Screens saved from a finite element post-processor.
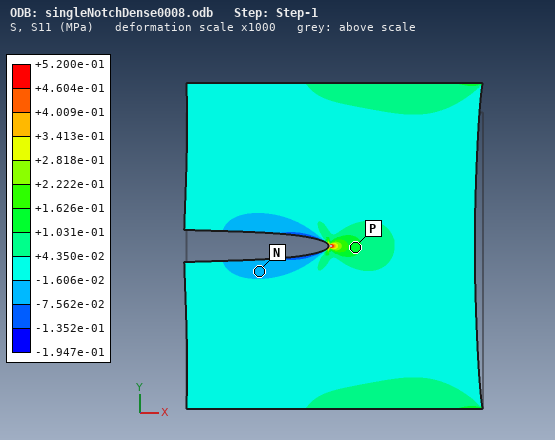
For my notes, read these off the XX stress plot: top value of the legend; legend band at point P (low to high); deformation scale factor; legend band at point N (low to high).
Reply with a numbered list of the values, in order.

1. +5.200e-01 MPa
2. +1.031e-01 to +1.626e-01 MPa
3. 1000
4. -7.562e-02 to -1.606e-02 MPa
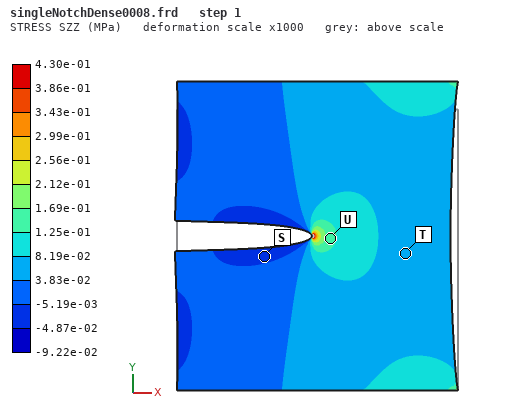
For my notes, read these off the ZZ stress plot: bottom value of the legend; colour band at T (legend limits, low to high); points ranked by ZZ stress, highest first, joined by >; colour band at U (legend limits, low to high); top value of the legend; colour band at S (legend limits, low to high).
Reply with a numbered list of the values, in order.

1. -9.22e-02 MPa
2. 3.83e-02 to 8.19e-02 MPa
3. U > T > S
4. 1.25e-01 to 1.69e-01 MPa
5. 4.30e-01 MPa
6. -4.87e-02 to -5.19e-03 MPa
